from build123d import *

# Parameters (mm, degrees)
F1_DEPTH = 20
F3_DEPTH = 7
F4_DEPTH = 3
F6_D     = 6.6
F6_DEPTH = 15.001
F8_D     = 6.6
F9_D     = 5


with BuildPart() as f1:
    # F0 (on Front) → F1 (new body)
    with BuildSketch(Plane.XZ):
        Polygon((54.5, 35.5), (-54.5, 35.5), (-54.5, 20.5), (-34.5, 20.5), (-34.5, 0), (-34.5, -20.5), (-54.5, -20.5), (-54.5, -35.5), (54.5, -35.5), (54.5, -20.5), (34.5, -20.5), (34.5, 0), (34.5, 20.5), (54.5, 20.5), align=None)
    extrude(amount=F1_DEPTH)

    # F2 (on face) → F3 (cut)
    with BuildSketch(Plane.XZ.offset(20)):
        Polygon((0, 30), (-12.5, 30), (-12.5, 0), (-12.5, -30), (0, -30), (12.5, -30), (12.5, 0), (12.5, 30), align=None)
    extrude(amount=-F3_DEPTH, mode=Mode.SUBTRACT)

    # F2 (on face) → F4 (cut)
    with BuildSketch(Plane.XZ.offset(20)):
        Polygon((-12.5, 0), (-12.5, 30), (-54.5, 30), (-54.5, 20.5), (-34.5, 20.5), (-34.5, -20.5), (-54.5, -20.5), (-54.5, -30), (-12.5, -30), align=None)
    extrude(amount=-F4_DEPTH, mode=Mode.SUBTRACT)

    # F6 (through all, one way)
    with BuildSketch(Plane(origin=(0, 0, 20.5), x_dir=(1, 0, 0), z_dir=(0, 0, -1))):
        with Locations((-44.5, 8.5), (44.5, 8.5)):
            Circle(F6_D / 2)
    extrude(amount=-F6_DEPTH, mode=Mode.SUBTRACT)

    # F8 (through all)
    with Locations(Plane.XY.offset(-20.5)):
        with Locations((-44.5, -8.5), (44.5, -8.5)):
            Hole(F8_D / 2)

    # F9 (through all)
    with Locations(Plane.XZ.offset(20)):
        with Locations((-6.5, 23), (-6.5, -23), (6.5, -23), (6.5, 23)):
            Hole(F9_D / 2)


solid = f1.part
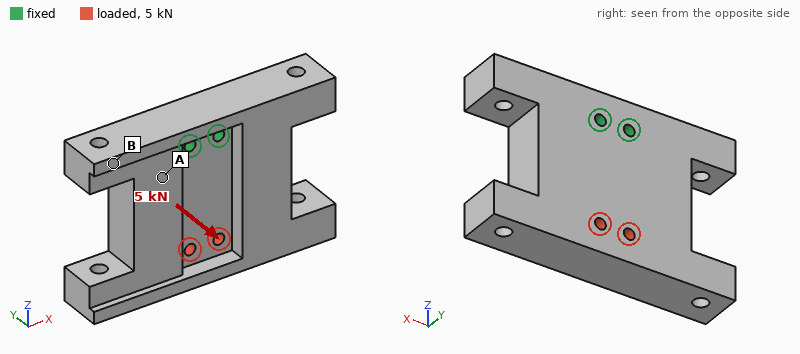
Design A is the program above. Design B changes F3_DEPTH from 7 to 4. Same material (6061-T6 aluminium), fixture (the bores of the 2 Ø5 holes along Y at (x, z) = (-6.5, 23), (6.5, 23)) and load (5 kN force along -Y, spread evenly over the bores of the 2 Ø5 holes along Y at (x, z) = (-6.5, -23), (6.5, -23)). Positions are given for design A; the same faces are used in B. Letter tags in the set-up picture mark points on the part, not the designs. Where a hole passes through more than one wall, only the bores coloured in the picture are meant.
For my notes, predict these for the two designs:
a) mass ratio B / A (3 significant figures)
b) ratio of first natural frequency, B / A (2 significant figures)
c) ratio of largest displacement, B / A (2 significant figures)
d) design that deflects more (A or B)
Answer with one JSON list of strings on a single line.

["1.04", "1.2", "0.70", "A"]
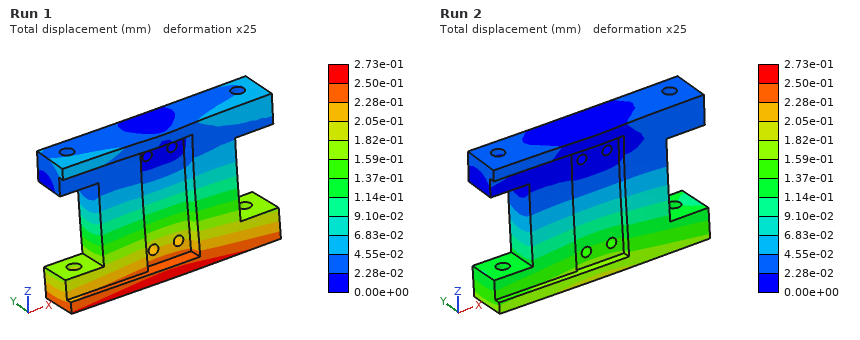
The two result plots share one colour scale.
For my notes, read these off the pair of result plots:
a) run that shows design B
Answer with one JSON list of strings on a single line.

["Run 2"]
